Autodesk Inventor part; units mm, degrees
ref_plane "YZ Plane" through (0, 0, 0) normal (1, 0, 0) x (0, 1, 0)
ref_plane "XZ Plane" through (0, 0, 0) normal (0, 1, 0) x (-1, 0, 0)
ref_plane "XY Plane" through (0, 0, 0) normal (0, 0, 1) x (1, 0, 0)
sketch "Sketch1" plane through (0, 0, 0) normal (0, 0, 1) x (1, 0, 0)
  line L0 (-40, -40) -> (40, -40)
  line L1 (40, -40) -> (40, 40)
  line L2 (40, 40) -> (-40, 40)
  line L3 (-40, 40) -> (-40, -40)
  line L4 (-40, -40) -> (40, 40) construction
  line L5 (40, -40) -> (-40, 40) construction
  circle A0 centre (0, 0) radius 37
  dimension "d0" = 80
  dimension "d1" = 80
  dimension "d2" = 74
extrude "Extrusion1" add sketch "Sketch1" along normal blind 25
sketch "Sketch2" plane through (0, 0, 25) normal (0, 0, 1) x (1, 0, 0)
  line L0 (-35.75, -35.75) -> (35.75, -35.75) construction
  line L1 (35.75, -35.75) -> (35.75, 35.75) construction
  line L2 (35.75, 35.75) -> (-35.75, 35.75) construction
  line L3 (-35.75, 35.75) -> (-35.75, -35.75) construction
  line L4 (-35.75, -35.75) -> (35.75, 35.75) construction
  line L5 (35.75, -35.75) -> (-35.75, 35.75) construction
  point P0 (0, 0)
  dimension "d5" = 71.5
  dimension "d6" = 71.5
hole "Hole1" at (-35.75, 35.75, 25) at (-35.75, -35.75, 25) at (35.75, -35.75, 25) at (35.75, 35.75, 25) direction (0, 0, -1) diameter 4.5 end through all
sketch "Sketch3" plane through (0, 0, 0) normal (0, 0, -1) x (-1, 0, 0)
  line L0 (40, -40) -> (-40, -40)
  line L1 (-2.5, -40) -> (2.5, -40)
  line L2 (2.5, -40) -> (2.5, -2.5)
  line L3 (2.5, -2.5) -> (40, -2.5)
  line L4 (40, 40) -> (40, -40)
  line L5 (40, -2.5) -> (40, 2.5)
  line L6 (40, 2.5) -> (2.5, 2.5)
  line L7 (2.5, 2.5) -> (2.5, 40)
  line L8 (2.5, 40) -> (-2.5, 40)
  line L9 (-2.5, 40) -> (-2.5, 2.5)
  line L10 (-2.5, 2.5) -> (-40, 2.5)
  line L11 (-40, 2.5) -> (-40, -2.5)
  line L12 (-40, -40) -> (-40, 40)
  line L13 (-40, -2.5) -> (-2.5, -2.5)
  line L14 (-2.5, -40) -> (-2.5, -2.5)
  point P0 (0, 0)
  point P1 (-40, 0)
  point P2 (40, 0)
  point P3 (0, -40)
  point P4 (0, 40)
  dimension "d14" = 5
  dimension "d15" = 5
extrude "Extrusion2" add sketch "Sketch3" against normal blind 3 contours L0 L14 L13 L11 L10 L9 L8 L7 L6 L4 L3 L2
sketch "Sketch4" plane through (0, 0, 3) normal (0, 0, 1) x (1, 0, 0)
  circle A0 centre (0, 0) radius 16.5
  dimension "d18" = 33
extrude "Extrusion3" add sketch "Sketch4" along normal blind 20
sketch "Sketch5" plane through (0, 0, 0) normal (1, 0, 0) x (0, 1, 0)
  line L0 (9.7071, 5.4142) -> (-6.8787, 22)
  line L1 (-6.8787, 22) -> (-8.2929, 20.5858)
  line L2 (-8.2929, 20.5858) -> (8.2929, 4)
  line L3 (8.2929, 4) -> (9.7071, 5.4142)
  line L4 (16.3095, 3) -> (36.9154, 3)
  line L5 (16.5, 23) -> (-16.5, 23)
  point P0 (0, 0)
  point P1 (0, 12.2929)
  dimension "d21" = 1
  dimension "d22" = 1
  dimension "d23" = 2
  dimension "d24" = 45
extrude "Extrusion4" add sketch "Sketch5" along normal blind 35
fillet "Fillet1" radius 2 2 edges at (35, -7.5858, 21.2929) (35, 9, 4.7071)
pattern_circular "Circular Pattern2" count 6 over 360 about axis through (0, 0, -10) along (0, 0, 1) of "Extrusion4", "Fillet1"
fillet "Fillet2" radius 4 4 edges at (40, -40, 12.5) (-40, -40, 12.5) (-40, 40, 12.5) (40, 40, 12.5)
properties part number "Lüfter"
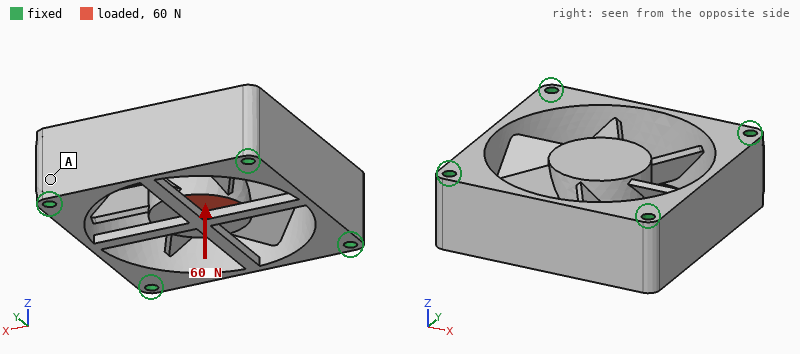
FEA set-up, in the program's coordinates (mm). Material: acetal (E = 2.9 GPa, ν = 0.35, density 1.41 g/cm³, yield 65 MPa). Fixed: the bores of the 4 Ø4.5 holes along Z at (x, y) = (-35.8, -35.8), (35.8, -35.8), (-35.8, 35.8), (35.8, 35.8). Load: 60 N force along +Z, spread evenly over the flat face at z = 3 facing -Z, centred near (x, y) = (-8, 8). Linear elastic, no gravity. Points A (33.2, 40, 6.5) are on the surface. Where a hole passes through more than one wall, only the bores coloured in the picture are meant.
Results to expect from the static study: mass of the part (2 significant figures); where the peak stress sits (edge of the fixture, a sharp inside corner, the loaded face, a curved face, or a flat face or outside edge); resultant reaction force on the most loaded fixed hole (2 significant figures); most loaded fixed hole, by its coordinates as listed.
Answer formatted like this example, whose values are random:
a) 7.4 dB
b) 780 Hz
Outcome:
a) 110 g
b) a flat face or outside edge
c) 23 N
d) (-35.8, 35.8)
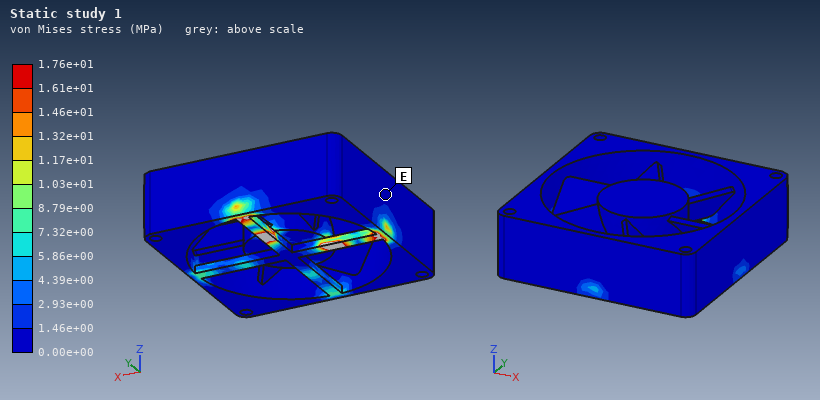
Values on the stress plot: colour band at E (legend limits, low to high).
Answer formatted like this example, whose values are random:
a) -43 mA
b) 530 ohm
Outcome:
a) 0.00e+00 to 1.46e+00 MPa
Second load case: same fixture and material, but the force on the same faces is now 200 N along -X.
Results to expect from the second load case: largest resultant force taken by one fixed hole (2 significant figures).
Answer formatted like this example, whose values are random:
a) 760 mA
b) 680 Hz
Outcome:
a) 90 N
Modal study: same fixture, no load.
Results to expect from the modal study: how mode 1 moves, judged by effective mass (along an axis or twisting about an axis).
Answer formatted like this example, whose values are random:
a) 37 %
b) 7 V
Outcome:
a) along Z
